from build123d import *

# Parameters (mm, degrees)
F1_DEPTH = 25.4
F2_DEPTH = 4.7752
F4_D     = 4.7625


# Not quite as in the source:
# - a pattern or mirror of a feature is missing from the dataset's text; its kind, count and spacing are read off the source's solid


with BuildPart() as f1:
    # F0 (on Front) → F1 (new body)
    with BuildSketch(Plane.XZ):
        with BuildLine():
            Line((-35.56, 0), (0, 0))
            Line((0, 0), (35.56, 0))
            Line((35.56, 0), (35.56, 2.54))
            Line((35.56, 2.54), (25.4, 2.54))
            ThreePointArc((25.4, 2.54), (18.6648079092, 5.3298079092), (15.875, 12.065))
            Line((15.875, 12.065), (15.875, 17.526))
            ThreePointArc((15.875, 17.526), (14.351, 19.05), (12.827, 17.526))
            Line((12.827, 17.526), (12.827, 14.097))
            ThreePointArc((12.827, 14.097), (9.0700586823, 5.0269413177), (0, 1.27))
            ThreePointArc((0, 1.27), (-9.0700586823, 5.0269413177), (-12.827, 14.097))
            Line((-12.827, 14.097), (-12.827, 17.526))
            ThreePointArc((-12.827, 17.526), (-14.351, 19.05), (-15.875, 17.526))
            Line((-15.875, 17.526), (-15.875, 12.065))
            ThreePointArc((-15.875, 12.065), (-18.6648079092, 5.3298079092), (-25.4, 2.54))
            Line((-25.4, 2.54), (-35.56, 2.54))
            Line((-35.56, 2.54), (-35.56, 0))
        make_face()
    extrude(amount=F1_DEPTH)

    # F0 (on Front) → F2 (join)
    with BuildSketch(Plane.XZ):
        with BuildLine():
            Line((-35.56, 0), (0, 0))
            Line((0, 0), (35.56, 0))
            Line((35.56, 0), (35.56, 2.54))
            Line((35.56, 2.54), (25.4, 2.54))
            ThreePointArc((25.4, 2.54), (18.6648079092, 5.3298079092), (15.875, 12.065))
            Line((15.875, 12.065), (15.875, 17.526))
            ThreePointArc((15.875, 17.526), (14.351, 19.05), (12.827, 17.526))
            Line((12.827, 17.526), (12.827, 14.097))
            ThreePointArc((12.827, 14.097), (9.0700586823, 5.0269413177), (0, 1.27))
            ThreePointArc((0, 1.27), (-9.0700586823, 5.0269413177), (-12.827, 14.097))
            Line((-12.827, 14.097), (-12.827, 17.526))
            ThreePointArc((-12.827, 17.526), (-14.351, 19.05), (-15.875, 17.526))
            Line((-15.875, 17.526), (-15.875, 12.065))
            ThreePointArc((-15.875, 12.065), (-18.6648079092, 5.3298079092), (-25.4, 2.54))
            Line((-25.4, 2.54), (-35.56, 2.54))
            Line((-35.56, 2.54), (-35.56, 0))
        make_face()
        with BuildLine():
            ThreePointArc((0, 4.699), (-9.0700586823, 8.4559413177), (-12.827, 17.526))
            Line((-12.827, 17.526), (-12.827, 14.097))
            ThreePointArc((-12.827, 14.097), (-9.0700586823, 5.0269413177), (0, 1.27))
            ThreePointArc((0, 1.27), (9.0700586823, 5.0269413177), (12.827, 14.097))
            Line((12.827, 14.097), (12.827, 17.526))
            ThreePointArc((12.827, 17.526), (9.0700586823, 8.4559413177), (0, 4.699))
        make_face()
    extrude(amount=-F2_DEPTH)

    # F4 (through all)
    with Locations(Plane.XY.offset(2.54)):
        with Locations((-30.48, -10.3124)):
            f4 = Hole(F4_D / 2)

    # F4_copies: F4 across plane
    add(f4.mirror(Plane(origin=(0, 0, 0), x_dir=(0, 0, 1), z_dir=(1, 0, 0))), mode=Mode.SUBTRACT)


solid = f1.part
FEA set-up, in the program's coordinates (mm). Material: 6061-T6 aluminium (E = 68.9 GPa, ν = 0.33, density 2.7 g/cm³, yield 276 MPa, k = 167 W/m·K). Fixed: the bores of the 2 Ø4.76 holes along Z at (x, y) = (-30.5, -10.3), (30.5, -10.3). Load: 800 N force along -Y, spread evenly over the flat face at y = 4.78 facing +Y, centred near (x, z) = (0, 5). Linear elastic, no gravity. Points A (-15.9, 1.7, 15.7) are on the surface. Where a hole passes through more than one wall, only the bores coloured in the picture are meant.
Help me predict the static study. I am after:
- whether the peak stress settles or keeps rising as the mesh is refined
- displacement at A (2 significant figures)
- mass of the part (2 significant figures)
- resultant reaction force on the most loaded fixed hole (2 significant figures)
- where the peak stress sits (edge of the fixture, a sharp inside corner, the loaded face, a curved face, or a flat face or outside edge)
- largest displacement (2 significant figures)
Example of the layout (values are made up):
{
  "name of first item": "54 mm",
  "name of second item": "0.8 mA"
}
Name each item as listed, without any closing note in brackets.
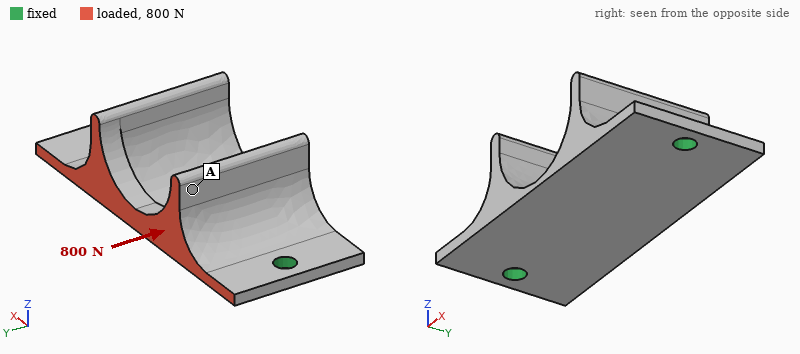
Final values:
{
  "whether the peak stress settles or keeps rising as the mesh is refined": "keeps rising",
  "displacement at A": "54 µm",
  "mass of the part": "30 g",
  "resultant reaction force on the most loaded fixed hole": "410 N",
  "where the peak stress sits": "edge of the fixture",
  "largest displacement": "66 µm"
}
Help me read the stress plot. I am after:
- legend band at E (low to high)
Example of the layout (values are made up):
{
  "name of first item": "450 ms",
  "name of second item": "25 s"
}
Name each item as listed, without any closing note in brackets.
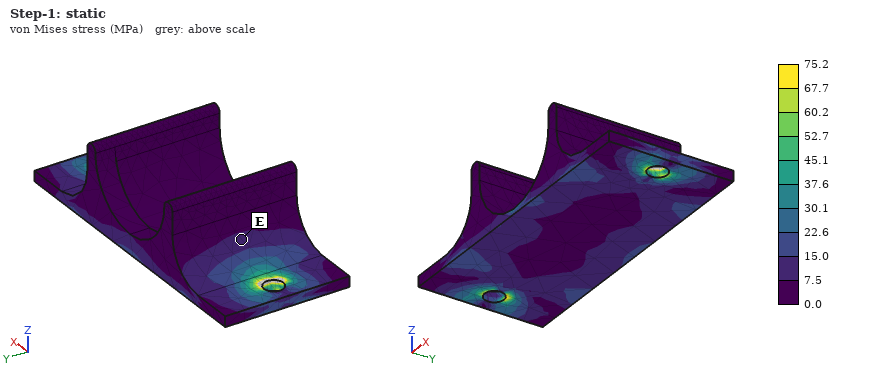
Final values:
{
  "legend band at E": "7.5 to 15.0 MPa"
}
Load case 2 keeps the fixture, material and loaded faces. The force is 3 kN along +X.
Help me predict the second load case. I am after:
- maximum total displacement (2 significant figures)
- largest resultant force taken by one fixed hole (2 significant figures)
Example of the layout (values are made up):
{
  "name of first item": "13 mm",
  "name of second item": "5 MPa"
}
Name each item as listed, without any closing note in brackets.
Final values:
{
  "maximum total displacement": "44 µm",
  "largest resultant force taken by one fixed hole": "1.7 kN"
}
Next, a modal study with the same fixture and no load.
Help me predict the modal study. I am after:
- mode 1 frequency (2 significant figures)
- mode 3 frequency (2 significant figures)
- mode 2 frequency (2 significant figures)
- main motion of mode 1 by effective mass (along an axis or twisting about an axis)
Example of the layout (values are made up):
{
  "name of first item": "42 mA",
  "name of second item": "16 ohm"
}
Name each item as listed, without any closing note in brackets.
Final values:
{
  "mode 1 frequency": "2800 Hz",
  "mode 3 frequency": "6300 Hz",
  "mode 2 frequency": "3000 Hz",
  "main motion of mode 1 by effective mass": "along Z"
}
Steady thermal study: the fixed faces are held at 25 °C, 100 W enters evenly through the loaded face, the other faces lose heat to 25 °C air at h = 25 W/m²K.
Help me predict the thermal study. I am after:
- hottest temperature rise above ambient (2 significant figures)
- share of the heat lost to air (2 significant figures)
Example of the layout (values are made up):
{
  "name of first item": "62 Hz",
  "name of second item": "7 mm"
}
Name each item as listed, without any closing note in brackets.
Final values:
{
  "hottest temperature rise above ambient": "77 K",
  "share of the heat lost to air": "7.0 %"
}
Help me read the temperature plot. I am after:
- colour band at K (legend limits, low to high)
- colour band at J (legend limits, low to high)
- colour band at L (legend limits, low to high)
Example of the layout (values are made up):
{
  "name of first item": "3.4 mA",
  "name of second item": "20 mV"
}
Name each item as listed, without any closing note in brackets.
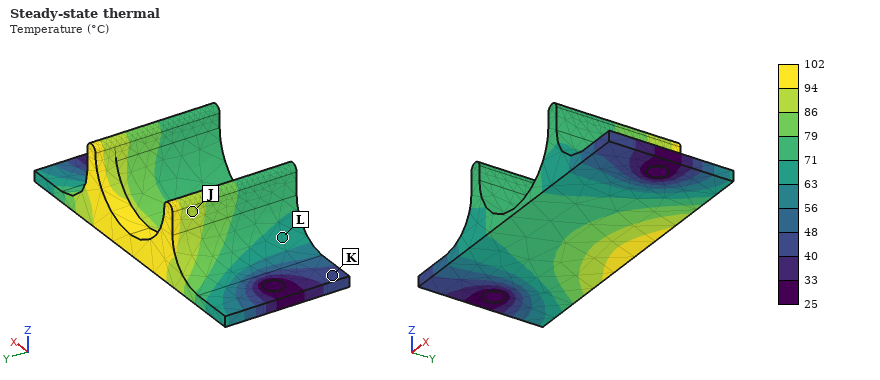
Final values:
{
  "colour band at K": "40 to 48 °C",
  "colour band at J": "86 to 94 °C",
  "colour band at L": "63 to 71 °C"
}
